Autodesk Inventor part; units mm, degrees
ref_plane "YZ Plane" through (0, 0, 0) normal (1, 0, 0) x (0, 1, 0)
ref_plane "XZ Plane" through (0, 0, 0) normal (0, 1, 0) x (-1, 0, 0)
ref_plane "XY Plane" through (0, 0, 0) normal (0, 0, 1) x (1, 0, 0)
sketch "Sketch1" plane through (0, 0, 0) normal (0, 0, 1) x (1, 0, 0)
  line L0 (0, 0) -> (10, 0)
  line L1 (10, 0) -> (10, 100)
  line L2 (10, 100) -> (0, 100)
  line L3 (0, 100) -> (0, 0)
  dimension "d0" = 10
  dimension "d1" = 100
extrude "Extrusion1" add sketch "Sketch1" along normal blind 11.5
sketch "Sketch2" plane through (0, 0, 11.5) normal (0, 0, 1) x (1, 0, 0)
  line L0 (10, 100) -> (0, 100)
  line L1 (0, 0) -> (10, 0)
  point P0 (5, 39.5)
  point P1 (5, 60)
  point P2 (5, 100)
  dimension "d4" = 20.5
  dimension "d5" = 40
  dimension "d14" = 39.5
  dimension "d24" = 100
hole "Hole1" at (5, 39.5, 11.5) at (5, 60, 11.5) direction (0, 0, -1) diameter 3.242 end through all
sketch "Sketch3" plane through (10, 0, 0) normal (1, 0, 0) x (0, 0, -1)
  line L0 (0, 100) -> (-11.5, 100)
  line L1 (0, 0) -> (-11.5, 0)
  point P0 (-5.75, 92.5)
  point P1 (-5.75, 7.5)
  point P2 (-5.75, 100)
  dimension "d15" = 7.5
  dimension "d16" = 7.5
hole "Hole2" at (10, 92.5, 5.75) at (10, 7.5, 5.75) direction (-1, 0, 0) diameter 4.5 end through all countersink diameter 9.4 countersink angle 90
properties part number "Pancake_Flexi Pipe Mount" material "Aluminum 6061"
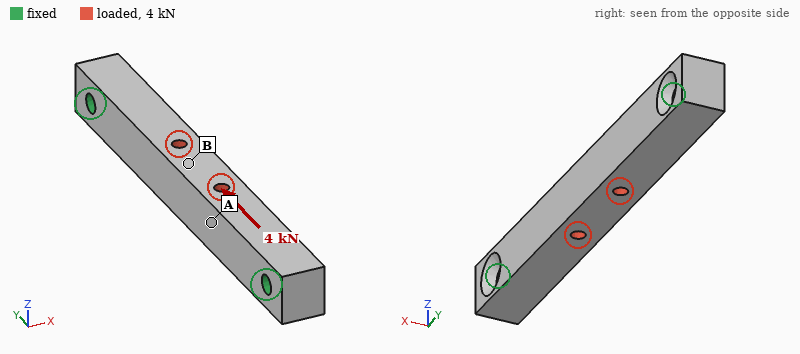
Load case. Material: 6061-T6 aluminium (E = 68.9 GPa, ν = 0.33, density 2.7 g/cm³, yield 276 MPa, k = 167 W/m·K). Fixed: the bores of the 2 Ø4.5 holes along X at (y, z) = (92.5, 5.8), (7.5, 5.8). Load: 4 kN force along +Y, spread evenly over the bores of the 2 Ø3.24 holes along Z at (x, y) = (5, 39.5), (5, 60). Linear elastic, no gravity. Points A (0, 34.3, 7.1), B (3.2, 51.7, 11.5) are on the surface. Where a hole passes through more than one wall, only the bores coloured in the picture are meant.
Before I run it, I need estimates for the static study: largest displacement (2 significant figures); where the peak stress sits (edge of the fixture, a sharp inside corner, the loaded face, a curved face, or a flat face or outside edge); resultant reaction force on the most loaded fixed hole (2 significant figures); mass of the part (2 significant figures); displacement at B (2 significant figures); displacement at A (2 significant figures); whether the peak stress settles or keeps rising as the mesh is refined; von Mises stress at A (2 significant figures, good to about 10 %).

9.5 µm
edge of the fixture
2.0 kN
29 g
8.9 µm
7.3 µm
keeps rising
18 MPa
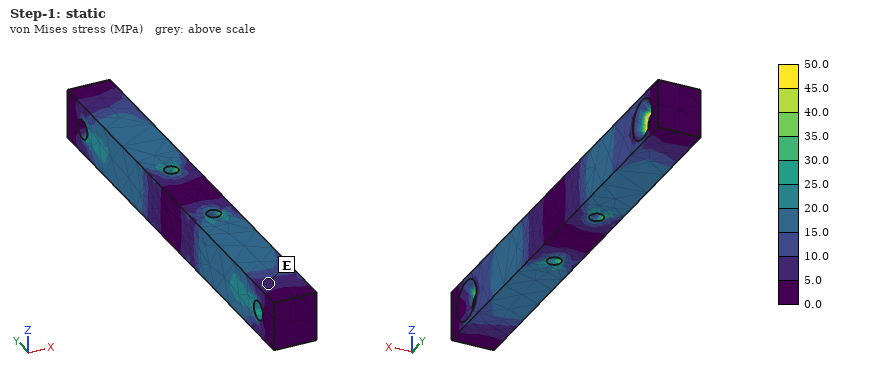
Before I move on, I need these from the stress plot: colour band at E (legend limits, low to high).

5.0 to 10.0 MPa
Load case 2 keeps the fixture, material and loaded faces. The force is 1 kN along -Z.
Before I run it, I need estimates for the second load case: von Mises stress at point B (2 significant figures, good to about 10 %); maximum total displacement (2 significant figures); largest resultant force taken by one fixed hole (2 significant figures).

30 MPa
49 µm
500 N
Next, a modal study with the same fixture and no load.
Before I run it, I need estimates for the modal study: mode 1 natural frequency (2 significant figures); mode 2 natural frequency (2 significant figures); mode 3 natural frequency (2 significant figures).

6400 Hz
6500 Hz
16 kHz
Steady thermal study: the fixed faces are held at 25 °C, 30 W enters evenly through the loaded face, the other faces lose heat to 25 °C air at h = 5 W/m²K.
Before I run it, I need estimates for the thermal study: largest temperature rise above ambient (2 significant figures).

26 K
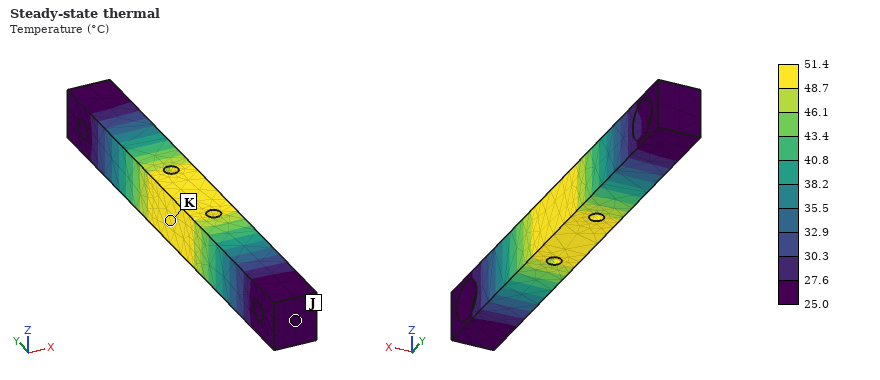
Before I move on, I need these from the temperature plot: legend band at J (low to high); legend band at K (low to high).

25.0 to 27.6 °C
48.7 to 51.4 °C
